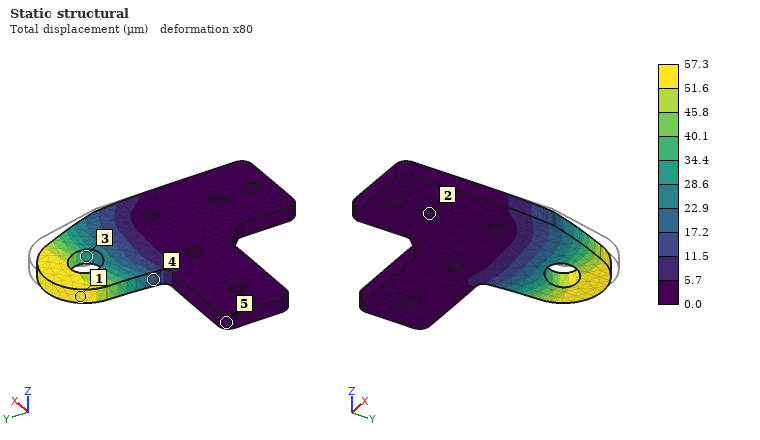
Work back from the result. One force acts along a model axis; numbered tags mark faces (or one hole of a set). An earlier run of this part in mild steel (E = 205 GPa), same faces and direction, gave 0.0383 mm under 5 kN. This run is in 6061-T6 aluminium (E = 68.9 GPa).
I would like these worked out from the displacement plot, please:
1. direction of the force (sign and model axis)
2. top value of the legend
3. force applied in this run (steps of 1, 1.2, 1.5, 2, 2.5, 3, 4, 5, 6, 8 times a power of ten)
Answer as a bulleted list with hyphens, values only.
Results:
- -X
- 57.3 µm
- 2.5 kN
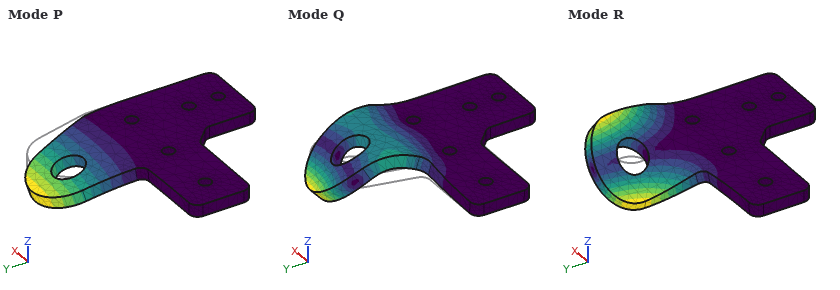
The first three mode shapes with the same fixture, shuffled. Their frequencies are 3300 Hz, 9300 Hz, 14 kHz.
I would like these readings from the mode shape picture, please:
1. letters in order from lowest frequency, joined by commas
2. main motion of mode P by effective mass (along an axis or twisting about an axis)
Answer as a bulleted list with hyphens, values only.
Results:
- P, R, Q
- along Z
